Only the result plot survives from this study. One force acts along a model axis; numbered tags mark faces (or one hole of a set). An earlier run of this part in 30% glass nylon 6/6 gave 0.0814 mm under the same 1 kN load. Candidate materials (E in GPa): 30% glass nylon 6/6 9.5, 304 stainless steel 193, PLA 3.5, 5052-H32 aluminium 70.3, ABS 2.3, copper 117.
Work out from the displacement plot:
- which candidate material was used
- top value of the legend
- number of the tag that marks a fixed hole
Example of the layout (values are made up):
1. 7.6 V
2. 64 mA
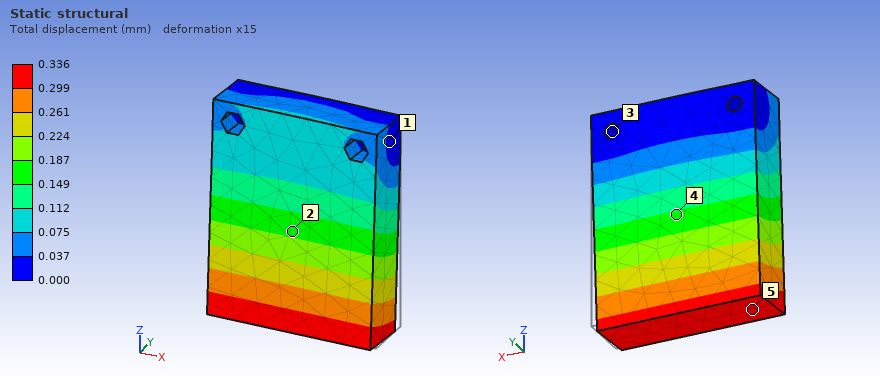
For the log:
1. ABS
2. 0.336 mm
3. 3
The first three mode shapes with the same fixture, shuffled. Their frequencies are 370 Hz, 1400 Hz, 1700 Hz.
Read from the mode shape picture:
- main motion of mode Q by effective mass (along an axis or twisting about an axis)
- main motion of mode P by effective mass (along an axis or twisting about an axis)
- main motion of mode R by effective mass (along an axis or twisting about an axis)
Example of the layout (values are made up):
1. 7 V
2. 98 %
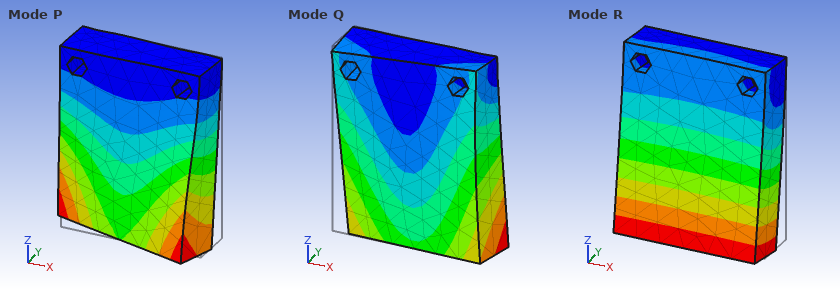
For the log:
1. along X
2. along X
3. along Y
